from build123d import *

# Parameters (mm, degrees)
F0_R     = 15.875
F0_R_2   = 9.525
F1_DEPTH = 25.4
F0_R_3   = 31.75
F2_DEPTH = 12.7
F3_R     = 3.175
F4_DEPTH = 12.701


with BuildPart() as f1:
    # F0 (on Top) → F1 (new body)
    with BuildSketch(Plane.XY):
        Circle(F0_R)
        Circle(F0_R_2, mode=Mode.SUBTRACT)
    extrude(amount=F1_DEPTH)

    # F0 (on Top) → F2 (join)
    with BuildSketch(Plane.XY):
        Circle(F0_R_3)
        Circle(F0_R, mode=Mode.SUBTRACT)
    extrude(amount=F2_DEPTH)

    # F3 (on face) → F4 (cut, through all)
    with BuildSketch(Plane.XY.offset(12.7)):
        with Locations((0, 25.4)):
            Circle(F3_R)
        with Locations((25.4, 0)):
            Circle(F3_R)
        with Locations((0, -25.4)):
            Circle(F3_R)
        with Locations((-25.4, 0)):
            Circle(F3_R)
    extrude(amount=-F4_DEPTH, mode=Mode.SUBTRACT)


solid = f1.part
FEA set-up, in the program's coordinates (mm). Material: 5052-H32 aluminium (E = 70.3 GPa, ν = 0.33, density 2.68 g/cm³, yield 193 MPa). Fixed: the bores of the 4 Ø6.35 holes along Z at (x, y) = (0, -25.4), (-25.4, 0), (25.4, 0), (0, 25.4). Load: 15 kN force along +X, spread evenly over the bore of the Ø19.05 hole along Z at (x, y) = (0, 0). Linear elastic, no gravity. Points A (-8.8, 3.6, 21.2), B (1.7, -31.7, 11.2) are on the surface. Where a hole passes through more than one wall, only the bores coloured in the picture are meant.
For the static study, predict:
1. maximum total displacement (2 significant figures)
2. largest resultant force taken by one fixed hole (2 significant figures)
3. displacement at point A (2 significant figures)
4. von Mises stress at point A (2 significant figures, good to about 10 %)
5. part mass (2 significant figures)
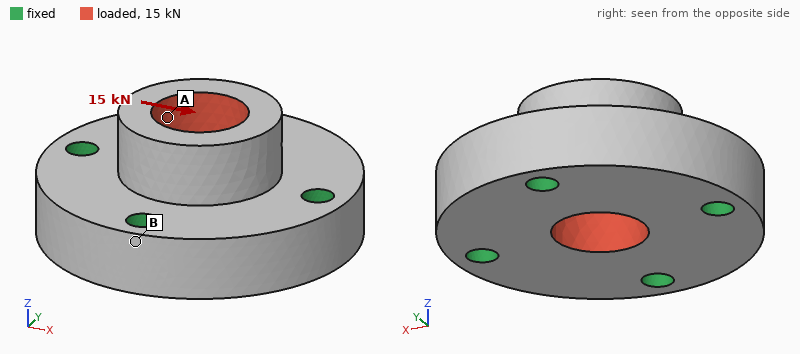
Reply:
19 µm
5.0 kN
14 µm
21 MPa
110 g
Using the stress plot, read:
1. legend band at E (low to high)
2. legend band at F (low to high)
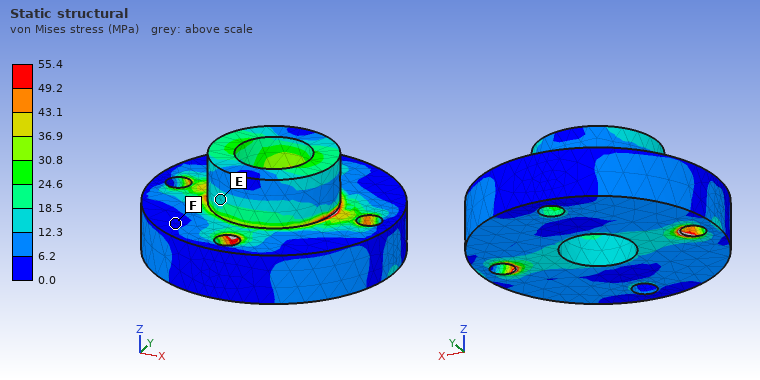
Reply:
12.3 to 18.5 MPa
0.0 to 6.2 MPa
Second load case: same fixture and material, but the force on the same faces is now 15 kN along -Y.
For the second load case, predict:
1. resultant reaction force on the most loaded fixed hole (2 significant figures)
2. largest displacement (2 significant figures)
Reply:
5.0 kN
18 µm
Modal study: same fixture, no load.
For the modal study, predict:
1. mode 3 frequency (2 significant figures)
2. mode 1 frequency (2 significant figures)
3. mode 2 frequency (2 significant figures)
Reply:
26 kHz
26 kHz
26 kHz
